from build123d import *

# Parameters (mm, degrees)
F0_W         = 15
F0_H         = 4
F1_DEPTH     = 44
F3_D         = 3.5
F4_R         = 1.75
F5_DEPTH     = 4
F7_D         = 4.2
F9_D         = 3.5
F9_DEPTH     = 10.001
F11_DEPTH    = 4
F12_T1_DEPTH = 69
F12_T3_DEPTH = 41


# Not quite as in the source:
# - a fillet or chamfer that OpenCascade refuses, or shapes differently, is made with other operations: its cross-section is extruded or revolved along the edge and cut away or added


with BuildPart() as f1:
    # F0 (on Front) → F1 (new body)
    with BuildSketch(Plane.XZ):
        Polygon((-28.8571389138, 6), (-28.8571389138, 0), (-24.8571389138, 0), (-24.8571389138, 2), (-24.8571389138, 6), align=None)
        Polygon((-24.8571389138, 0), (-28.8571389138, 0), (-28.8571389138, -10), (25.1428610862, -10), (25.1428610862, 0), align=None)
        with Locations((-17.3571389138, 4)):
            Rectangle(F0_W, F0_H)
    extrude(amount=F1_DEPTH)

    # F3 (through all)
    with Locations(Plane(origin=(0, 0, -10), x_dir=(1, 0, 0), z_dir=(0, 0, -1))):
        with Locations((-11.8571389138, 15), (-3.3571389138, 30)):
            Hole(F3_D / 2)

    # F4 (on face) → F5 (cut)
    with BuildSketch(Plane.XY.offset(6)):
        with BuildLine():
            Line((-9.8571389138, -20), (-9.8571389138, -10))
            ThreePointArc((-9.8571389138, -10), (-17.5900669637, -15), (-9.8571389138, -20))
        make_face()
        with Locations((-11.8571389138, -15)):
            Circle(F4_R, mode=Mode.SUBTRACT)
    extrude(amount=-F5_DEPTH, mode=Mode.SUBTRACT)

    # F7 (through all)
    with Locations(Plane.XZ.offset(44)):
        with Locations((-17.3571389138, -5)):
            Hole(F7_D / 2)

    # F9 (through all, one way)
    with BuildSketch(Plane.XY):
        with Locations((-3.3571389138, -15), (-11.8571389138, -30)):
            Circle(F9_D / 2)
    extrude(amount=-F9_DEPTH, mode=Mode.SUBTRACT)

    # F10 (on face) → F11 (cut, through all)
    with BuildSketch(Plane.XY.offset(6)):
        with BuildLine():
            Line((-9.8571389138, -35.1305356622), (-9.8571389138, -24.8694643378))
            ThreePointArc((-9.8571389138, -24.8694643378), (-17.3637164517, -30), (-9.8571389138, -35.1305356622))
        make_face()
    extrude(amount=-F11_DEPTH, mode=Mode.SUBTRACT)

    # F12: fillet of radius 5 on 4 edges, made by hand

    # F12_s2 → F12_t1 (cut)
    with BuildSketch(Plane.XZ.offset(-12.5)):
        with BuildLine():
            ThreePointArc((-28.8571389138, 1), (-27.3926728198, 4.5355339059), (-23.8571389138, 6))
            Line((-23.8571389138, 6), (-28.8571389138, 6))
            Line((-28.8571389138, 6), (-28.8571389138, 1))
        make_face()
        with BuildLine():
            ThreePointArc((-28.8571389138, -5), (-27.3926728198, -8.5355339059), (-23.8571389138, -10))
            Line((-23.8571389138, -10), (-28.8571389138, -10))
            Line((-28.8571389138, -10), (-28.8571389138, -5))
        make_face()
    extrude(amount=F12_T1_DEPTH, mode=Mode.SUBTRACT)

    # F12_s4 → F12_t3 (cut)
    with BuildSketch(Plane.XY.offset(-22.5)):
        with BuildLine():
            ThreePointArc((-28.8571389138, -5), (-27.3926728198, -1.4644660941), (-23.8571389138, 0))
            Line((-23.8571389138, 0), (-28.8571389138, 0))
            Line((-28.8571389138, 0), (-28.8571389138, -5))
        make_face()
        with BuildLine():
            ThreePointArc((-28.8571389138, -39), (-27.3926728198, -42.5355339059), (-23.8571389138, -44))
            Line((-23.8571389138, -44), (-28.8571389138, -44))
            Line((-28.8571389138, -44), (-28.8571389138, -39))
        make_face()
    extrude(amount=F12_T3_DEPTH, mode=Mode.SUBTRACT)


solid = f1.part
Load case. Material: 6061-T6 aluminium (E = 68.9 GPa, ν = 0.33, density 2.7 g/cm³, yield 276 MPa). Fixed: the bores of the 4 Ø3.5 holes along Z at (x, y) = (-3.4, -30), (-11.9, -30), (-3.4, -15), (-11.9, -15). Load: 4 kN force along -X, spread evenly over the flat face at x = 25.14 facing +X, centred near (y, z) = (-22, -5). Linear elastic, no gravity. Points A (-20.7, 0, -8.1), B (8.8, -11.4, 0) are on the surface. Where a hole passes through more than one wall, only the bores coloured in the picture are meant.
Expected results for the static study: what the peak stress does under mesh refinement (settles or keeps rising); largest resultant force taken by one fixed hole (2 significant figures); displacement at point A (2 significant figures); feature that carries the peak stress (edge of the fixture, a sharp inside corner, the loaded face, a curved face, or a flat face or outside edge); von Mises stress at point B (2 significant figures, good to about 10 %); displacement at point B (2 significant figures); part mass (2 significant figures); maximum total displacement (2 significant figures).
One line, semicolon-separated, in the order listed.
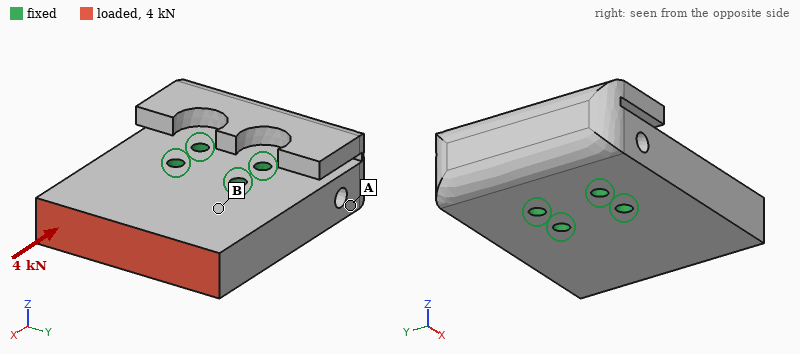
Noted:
keeps rising; 1.5 kN; 1.3 µm; edge of the fixture; 10 MPa; 2.5 µm; 68 g; 5.3 µm
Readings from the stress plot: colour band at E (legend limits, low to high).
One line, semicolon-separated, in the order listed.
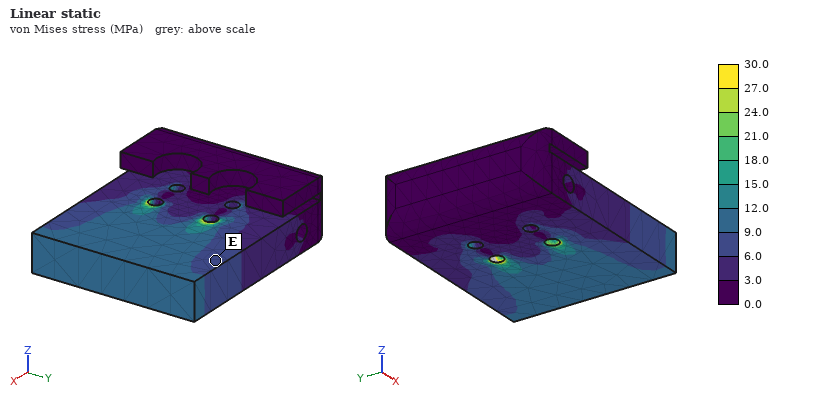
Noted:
6.0 to 9.0 MPa
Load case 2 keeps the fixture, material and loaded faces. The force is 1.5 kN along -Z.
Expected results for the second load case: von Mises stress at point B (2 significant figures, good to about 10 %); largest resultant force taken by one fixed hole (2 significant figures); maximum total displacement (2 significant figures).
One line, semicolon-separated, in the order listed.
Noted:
31 MPa; 1.3 kN; 59 µm
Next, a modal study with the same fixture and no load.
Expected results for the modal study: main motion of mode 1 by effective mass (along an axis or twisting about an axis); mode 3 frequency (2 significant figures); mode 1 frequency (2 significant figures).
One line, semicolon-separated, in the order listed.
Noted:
along Z; 9800 Hz; 8400 Hz
